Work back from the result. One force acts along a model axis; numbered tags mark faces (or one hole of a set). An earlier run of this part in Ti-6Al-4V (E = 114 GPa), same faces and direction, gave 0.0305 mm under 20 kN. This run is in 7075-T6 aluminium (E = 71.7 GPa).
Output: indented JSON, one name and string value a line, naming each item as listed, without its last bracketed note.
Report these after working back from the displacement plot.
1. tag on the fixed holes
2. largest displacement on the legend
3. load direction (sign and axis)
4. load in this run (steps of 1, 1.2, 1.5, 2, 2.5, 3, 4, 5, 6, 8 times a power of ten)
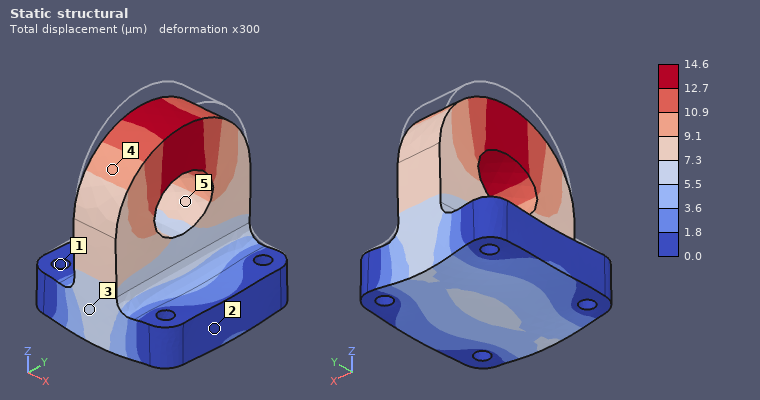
{
  "tag on the fixed holes": "1",
  "largest displacement on the legend": "14.6 µm",
  "load direction": "-Z",
  "load in this run": "6 kN"
}
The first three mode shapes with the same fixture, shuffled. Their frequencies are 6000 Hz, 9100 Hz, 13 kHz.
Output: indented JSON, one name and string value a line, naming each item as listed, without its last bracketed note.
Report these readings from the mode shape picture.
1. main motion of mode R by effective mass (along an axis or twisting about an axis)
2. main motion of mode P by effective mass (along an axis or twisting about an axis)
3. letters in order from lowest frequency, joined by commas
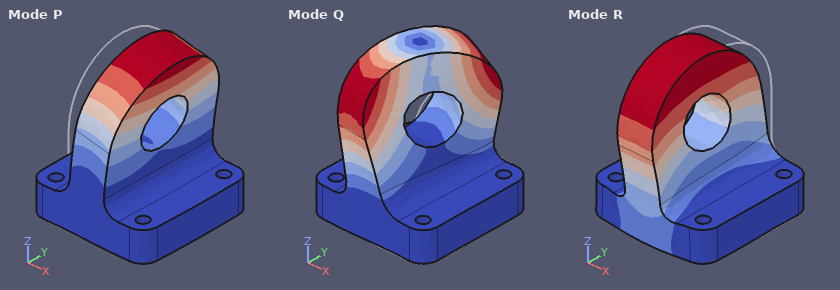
{
  "main motion of mode R by effective mass": "along Y",
  "main motion of mode P by effective mass": "along X",
  "letters in order from lowest frequency, joined by commas": "P, R, Q"
}
